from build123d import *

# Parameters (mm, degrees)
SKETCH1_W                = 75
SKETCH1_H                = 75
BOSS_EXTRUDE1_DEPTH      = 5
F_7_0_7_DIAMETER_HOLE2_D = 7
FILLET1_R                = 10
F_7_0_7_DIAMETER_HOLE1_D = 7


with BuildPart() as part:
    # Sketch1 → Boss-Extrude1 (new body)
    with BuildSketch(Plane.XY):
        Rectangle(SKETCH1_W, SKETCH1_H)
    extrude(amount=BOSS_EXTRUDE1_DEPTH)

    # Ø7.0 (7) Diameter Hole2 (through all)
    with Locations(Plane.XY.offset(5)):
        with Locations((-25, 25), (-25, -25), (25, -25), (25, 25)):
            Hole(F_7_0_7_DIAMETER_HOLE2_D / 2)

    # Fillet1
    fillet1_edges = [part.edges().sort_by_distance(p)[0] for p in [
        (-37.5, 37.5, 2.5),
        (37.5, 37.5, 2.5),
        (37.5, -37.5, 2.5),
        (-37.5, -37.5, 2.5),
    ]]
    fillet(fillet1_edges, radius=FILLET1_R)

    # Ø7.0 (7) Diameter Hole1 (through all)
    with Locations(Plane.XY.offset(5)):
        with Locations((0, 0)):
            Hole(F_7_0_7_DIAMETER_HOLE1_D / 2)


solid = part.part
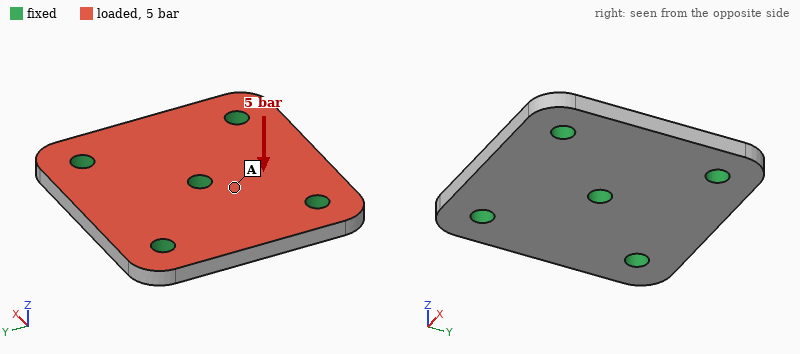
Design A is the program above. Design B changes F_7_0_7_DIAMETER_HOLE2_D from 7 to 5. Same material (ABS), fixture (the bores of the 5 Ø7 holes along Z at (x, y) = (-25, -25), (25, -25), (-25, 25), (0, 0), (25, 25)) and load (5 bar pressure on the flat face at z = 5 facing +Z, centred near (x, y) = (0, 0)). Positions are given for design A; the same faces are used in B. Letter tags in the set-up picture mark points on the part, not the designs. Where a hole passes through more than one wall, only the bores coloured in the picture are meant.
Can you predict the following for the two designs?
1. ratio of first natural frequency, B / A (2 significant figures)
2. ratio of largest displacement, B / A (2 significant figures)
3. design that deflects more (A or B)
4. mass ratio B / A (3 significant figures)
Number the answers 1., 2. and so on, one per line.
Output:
1. 0.89
2. 1.2
3. B
4. 1.01
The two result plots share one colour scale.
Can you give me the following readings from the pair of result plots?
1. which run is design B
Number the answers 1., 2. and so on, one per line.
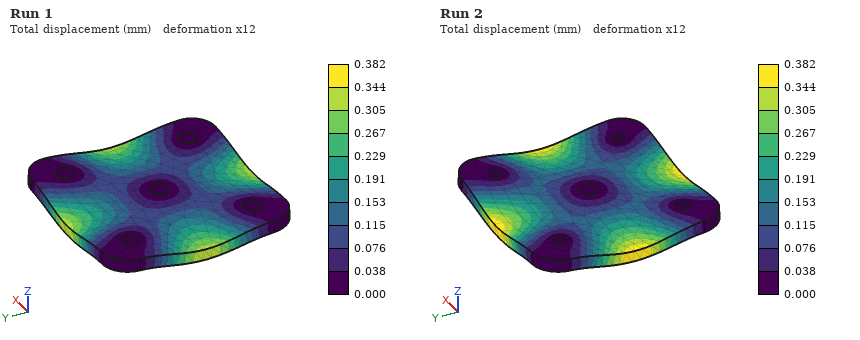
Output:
1. Run 2
